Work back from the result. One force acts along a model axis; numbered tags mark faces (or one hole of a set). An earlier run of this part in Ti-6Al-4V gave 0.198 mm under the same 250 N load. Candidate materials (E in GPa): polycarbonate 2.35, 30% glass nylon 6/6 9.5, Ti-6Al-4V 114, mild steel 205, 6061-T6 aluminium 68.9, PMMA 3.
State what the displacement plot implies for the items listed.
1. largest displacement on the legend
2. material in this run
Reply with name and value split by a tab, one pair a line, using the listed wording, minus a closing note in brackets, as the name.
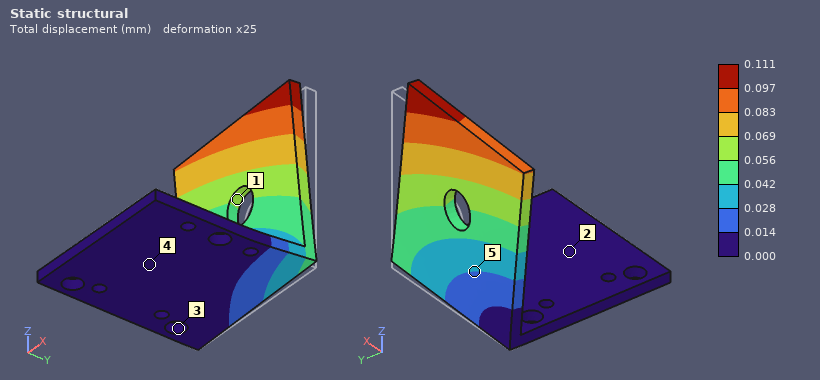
largest displacement on the legend	0.111 mm
material in this run	mild steel
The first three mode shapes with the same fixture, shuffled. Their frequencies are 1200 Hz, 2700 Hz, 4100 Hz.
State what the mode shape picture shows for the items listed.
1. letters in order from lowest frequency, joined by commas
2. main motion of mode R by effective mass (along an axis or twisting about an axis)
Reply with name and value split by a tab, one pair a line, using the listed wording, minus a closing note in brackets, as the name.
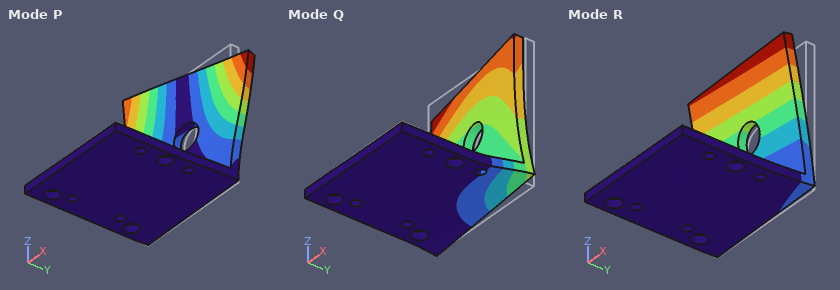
letters in order from lowest frequency, joined by commas	R, Q, P
main motion of mode R by effective mass	along Y
